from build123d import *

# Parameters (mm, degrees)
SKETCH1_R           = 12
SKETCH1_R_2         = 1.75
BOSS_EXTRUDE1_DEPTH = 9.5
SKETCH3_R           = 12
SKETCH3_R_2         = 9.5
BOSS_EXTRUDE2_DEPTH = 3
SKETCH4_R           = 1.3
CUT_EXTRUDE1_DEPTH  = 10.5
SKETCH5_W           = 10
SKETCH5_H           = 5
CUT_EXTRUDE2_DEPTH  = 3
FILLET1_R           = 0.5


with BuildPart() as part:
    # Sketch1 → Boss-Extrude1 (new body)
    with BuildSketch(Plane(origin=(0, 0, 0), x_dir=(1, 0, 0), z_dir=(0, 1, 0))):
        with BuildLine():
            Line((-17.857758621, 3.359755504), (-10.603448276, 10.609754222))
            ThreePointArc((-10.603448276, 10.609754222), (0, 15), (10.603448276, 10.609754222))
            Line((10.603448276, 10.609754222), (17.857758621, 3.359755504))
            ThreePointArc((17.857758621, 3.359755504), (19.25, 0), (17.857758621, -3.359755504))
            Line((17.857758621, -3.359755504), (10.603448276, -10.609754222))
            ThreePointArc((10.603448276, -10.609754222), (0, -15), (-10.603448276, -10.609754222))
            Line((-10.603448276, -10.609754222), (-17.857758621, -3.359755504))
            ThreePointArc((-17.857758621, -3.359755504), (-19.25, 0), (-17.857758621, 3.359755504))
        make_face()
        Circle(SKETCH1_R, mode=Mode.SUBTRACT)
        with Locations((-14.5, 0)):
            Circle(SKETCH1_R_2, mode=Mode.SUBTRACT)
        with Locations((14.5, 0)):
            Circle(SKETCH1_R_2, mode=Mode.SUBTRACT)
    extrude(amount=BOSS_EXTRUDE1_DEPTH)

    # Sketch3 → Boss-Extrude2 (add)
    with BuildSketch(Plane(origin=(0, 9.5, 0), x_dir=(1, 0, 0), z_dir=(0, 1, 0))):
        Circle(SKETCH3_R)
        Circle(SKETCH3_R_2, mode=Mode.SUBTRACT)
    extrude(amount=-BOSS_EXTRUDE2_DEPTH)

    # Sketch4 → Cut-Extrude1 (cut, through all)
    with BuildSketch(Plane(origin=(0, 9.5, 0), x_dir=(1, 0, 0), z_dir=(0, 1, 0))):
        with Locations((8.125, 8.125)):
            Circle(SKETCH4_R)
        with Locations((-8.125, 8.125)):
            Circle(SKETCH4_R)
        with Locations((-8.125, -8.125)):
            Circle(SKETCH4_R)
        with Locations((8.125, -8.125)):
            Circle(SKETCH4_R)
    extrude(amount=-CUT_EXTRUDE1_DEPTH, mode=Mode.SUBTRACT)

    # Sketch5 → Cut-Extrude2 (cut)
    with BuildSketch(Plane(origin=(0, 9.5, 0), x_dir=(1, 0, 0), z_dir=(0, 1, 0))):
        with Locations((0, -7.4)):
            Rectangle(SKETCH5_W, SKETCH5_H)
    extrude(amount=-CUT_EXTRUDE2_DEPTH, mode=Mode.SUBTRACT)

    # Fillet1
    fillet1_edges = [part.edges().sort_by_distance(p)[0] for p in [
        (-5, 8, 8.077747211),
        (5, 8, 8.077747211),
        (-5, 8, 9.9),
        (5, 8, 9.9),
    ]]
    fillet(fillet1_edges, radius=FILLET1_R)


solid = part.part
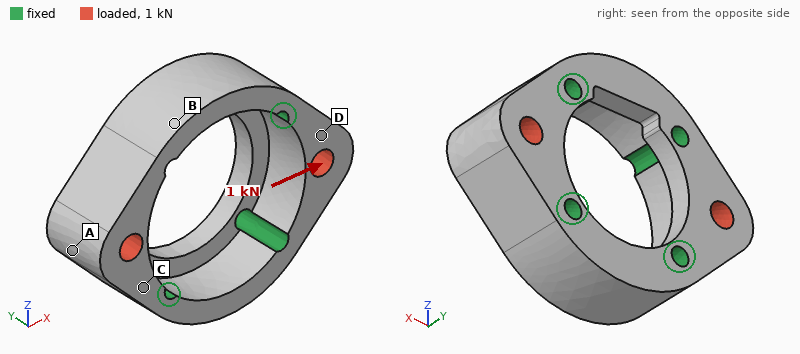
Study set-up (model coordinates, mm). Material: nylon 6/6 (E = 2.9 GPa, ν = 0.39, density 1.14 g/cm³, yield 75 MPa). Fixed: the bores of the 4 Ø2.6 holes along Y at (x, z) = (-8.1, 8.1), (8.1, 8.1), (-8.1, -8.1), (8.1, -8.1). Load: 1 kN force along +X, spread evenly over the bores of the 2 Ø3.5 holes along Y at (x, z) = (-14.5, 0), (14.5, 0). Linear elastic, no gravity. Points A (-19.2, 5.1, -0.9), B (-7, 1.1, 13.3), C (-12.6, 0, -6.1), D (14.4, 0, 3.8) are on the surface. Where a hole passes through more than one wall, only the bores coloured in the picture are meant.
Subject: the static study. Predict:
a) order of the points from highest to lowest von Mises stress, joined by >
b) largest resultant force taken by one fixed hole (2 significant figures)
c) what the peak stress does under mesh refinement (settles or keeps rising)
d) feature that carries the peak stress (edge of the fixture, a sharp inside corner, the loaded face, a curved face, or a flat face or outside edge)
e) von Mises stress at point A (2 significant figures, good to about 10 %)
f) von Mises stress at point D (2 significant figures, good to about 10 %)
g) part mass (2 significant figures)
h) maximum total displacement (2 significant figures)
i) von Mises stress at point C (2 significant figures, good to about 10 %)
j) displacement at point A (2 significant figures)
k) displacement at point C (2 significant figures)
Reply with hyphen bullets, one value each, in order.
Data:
- C > D > A > B
- 320 N
- keeps rising
- edge of the fixture
- 4.3 MPa
- 9.4 MPa
- 3.9 g
- 86 µm
- 12 MPa
- 44 µm
- 26 µm
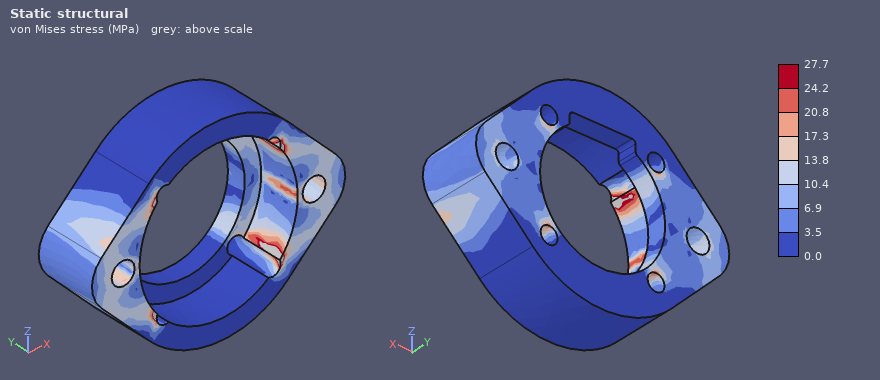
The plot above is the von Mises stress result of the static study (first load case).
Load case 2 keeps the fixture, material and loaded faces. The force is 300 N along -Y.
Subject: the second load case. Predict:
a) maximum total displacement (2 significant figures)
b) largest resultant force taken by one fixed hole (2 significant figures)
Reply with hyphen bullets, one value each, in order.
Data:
- 44 µm
- 75 N
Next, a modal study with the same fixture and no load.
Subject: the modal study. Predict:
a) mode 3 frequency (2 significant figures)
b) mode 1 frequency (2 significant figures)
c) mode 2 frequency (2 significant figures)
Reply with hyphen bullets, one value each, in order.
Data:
- 18 kHz
- 12 kHz
- 12 kHz
